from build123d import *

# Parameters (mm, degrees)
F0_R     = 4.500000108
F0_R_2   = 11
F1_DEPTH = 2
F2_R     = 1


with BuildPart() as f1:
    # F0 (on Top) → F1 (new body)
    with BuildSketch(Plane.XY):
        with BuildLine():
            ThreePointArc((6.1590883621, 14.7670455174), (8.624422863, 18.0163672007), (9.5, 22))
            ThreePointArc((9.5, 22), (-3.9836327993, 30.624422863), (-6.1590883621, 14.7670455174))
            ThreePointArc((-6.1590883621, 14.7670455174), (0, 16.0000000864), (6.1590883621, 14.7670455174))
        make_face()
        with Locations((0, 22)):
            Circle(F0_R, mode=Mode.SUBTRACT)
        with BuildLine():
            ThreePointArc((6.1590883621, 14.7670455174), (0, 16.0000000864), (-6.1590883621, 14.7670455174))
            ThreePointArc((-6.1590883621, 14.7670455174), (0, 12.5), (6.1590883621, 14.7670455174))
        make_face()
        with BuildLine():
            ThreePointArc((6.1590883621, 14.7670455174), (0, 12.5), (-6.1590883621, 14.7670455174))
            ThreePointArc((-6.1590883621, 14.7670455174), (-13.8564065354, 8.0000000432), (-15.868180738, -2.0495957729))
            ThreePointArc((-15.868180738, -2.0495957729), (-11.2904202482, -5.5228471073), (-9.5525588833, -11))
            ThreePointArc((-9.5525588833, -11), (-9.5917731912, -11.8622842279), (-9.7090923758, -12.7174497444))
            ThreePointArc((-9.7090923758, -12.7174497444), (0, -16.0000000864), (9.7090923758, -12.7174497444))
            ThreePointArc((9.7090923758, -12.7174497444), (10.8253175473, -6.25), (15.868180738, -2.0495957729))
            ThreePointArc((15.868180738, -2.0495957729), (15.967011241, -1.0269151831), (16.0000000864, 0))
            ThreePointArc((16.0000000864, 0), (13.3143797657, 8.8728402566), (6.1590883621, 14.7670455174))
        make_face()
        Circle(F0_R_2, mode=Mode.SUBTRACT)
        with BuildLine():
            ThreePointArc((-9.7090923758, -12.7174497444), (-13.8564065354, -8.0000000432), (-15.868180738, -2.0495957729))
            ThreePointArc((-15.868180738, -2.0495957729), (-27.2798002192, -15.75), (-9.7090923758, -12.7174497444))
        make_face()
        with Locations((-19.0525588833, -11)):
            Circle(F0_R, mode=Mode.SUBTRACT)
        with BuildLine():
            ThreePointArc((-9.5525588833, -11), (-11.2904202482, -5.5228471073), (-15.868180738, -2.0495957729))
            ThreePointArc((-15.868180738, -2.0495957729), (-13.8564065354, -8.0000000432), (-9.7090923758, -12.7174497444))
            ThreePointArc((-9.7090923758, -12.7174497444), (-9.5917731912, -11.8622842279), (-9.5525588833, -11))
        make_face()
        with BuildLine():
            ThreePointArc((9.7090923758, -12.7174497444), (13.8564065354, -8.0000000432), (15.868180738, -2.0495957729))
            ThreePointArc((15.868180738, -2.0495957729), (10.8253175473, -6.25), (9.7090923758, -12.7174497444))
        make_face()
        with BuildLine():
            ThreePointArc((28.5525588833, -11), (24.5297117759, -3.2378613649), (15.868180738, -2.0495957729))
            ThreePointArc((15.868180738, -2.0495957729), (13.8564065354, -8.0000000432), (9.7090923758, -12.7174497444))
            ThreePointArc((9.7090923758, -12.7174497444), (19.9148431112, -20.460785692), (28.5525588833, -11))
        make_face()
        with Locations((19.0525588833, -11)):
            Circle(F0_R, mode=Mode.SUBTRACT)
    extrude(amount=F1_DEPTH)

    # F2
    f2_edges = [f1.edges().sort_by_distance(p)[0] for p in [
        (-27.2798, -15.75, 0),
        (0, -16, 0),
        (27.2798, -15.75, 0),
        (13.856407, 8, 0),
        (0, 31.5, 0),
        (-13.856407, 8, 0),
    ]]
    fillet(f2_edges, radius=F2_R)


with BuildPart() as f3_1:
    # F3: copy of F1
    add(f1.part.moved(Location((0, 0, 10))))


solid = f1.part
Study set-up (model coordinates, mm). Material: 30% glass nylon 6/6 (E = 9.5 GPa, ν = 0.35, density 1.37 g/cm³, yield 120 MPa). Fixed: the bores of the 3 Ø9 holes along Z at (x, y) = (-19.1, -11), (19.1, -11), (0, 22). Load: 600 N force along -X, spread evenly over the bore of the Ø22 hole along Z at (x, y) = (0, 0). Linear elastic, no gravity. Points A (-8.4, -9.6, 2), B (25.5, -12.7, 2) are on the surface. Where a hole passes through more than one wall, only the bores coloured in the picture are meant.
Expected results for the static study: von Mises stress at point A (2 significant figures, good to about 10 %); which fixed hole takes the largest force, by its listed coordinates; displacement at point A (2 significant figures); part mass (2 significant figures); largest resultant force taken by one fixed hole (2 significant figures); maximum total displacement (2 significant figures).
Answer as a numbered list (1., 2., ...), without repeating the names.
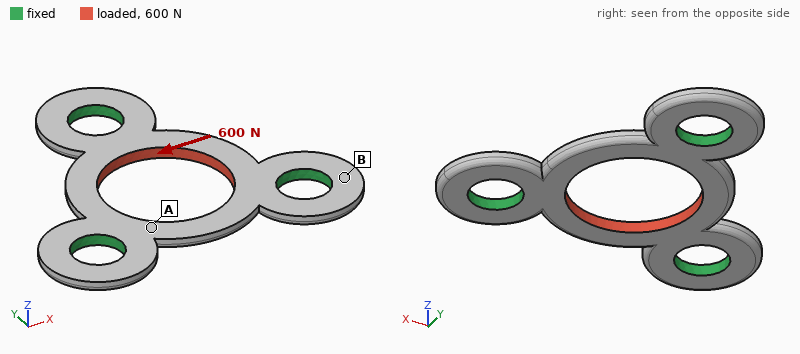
1. 7.7 MPa
2. (0, 22)
3. 8.6 µm
4. 2.7 g
5. 230 N
6. 41 µm
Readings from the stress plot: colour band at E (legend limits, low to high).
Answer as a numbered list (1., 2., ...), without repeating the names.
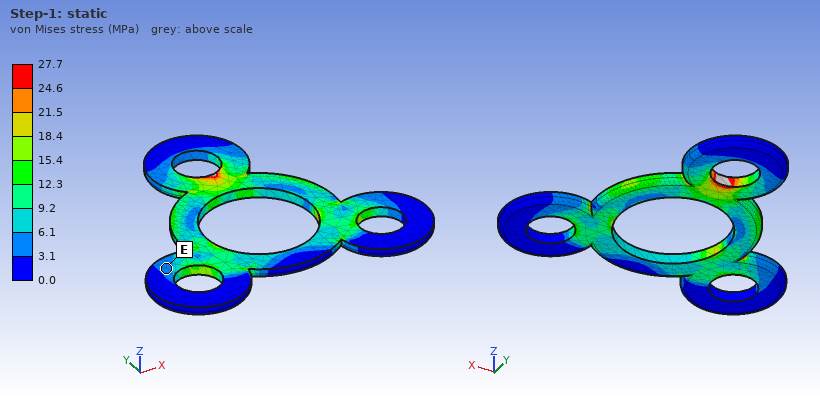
1. 3.1 to 6.1 MPa
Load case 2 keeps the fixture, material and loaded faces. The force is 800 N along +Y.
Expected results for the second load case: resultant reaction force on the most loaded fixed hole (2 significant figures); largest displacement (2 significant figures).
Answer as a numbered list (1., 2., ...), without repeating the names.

1. 290 N
2. 62 µm
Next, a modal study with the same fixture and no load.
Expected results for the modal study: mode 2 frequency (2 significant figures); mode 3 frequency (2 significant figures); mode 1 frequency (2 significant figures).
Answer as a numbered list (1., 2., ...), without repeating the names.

1. 6600 Hz
2. 6900 Hz
3. 6600 Hz
